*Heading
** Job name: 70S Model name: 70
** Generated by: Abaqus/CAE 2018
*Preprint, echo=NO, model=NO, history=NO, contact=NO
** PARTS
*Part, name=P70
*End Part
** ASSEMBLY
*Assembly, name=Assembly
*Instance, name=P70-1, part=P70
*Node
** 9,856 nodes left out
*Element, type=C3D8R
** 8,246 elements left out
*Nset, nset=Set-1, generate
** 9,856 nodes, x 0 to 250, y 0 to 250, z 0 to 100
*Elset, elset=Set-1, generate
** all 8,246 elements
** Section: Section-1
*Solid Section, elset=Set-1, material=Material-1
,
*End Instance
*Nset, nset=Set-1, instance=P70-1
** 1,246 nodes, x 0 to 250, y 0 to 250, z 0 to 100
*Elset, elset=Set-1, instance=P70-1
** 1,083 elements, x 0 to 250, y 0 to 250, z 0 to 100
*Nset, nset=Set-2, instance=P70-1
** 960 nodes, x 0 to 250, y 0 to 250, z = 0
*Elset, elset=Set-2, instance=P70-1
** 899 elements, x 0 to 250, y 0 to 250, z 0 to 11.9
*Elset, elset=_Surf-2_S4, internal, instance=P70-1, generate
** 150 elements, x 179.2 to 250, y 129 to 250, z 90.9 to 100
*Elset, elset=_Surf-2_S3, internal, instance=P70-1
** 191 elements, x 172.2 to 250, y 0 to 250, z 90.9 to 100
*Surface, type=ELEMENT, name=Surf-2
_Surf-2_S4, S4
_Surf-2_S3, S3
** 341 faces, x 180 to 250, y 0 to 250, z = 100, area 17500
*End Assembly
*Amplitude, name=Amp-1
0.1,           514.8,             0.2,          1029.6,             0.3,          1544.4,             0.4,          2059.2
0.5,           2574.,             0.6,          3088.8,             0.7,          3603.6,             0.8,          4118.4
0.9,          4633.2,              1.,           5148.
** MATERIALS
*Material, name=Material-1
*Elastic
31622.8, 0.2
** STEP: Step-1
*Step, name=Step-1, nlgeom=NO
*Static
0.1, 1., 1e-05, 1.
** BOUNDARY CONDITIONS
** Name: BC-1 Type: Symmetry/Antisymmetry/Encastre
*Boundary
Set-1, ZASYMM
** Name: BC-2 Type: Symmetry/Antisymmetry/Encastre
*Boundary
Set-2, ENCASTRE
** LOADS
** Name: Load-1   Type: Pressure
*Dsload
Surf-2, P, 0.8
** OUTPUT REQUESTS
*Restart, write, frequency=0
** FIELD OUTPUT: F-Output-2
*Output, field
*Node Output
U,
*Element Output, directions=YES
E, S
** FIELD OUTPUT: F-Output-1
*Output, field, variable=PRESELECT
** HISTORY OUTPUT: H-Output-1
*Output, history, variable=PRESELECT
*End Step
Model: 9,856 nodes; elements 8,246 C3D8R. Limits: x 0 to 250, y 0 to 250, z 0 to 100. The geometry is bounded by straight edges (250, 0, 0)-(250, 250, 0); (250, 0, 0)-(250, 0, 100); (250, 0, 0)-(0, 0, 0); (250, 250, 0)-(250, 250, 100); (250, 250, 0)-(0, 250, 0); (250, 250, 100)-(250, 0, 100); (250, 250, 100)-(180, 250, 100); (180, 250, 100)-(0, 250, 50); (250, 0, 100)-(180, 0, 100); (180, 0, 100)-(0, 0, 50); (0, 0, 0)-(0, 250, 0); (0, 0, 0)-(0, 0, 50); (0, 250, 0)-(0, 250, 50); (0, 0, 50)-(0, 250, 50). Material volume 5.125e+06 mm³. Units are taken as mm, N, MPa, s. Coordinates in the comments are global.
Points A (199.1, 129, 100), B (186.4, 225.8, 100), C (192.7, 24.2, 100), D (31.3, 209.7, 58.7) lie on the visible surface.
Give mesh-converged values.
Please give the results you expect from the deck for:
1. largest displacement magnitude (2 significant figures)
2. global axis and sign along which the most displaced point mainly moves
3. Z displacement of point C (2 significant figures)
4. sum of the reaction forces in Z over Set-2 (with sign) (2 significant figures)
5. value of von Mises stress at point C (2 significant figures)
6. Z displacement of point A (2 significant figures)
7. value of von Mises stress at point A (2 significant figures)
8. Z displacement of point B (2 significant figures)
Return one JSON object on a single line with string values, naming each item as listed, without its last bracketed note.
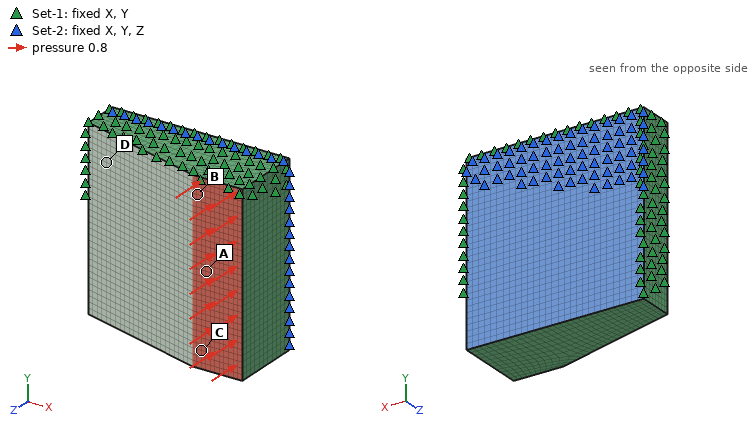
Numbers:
{"largest displacement magnitude": "0.0022 mm", "global axis and sign along which the most displaced point mainly moves": "-Z", "Z displacement of point C": "-0.0017 mm", "sum of the reaction forces in Z over Set-2 (with sign)": "14000 N", "value of von Mises stress at point C": "0.51 MPa", "Z displacement of point A": "-0.0018 mm", "value of von Mises stress at point A": "0.47 MPa", "Z displacement of point B": "-0.0015 mm"}
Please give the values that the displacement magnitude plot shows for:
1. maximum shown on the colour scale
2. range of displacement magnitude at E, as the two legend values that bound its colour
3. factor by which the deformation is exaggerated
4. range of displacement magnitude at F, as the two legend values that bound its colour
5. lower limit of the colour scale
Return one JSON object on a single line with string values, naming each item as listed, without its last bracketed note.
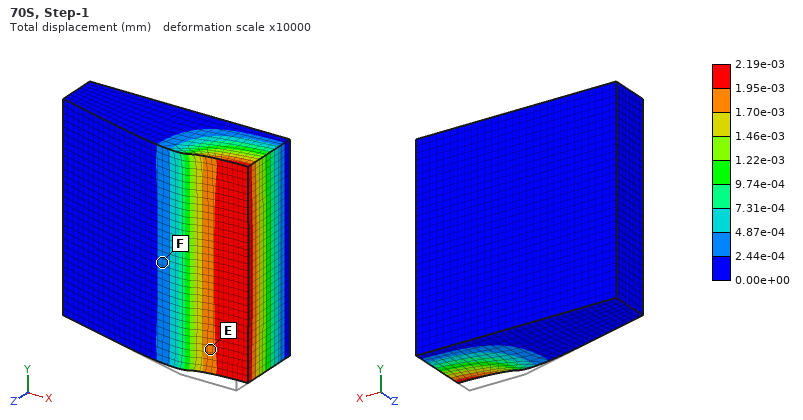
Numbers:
{"maximum shown on the colour scale": "2.19e-03 mm", "range of displacement magnitude at E, as the two legend values that bound its colour": "1.70e-03 to 1.95e-03 mm", "factor by which the deformation is exaggerated": "10000", "range of displacement magnitude at F, as the two legend values that bound its colour": "2.44e-04 to 4.87e-04 mm", "lower limit of the colour scale": "0.00e+00 mm"}
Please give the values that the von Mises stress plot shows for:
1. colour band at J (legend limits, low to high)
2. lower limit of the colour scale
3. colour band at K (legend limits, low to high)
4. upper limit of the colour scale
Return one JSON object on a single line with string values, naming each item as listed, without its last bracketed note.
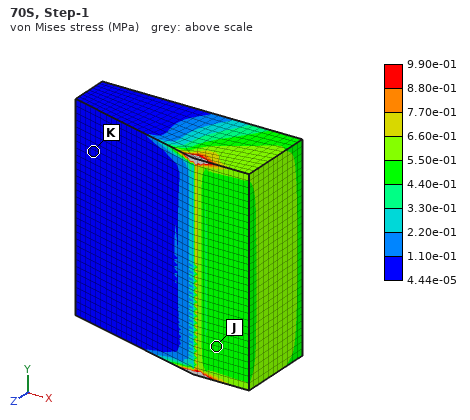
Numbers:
{"colour band at J": "4.40e-01 to 5.50e-01 MPa", "lower limit of the colour scale": "4.44e-05 MPa", "colour band at K": "4.44e-05 to 1.10e-01 MPa", "upper limit of the colour scale": "9.90e-01 MPa"}
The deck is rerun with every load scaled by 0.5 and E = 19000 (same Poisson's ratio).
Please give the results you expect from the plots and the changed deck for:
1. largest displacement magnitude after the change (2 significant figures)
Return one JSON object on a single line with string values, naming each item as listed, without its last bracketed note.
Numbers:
{"largest displacement magnitude after the change": "0.0018 mm"}
